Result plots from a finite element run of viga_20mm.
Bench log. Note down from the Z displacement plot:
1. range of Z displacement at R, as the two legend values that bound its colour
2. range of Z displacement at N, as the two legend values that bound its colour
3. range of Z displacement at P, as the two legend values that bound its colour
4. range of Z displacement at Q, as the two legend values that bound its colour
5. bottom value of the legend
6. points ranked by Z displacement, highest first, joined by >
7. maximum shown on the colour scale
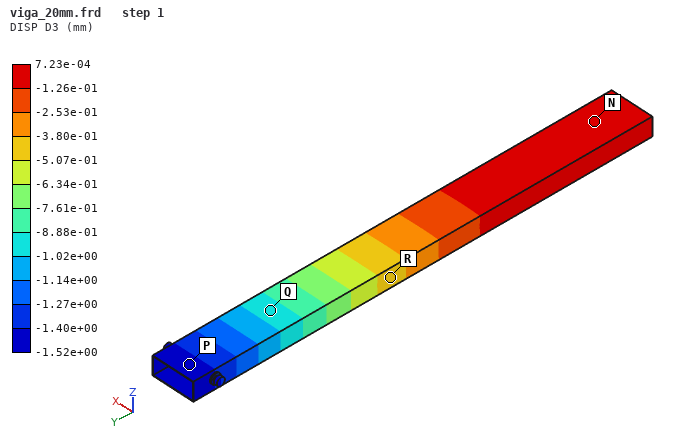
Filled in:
-5.07e-01 to -3.80e-01 mm
-1.26e-01 to 7.23e-04 mm
-1.52e+00 to -1.40e+00 mm
-1.02e+00 to -8.88e-01 mm
-1.52e+00 mm
N > R > Q > P
7.23e-04 mm
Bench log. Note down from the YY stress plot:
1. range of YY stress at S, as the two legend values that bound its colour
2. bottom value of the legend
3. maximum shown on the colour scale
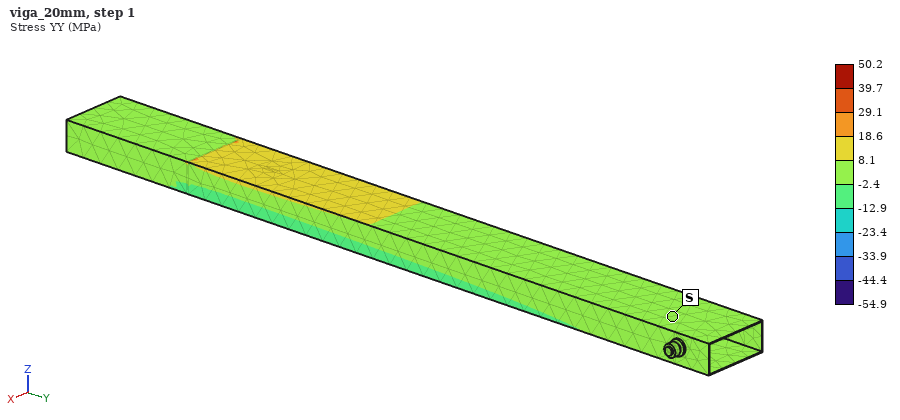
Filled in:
-2.4 to 8.1 MPa
-54.9 MPa
50.2 MPa
